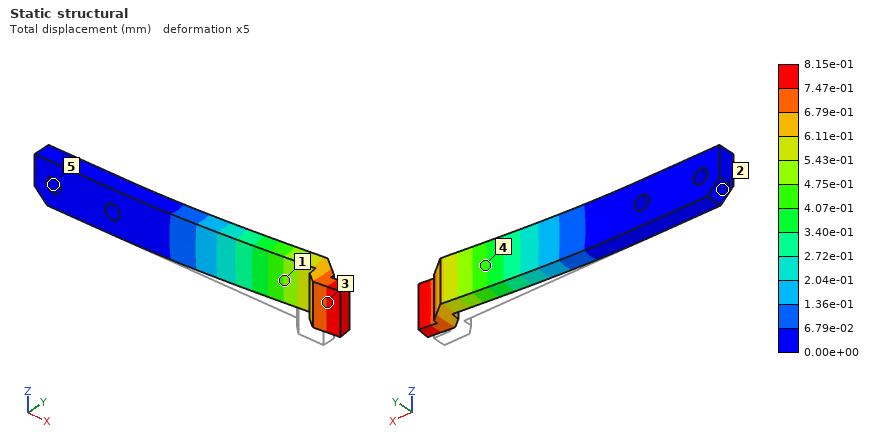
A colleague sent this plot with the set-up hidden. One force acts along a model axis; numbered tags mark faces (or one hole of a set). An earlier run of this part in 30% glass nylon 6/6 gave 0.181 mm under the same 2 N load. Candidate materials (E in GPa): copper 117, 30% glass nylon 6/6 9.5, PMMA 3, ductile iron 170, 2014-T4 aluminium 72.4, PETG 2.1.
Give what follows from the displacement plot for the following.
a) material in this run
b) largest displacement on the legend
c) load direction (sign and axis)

PETG
8.15e-01 mm
+Y
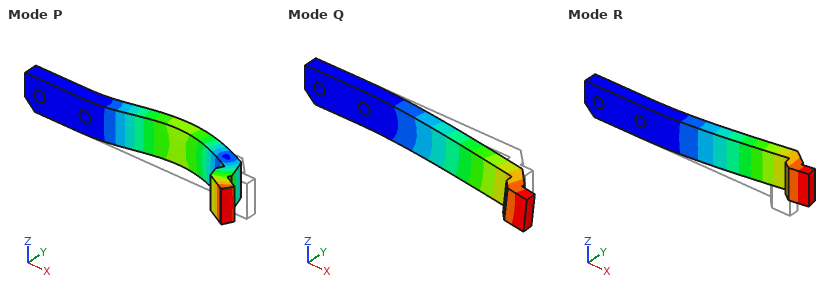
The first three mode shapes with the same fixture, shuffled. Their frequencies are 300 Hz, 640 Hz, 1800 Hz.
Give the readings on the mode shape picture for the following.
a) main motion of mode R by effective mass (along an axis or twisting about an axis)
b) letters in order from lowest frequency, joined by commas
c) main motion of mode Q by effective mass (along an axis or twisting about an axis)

along Y
R, Q, P
along Z
